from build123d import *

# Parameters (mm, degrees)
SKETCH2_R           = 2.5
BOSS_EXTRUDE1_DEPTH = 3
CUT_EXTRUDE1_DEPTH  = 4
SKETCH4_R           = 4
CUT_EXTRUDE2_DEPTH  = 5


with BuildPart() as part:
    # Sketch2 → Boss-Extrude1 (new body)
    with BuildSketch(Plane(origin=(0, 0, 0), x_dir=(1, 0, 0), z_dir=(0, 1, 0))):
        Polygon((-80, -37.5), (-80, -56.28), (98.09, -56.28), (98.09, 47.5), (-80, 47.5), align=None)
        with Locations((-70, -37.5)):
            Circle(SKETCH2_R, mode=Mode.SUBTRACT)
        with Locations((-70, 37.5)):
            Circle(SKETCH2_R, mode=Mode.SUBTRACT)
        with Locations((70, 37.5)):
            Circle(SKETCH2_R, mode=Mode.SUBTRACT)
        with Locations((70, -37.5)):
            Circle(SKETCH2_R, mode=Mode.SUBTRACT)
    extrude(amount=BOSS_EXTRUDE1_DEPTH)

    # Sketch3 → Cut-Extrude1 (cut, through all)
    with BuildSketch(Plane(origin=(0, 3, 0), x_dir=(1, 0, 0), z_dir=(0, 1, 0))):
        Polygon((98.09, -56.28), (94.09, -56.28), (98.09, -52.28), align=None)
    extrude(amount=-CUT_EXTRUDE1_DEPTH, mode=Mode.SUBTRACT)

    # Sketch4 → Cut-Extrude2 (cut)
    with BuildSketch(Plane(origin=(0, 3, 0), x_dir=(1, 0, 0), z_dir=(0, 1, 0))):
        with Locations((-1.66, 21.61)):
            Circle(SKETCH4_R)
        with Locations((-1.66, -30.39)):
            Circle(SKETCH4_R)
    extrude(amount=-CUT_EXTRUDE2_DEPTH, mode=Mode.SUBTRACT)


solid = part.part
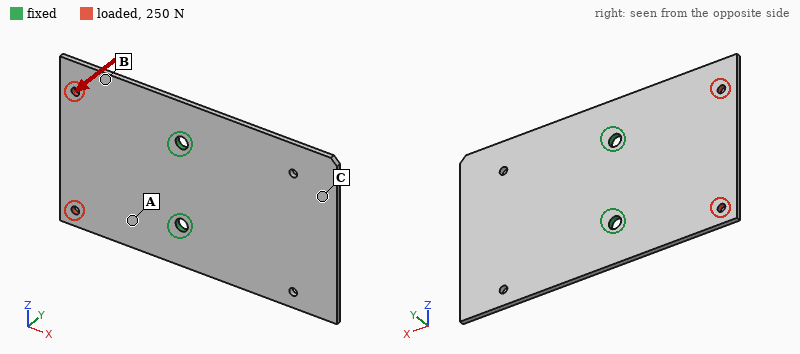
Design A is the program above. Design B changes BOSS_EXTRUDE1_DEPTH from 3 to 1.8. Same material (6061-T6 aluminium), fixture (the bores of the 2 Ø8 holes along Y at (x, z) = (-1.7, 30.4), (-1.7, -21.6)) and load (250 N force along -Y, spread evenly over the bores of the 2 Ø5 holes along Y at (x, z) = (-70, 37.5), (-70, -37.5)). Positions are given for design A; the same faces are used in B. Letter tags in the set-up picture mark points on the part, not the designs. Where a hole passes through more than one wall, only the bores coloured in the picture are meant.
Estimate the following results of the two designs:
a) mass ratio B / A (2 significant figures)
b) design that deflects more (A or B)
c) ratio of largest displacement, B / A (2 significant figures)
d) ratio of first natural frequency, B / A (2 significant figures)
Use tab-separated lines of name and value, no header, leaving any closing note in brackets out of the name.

mass ratio B / A	0.60
design that deflects more	B
ratio of largest displacement, B / A	4.6
ratio of first natural frequency, B / A	0.60
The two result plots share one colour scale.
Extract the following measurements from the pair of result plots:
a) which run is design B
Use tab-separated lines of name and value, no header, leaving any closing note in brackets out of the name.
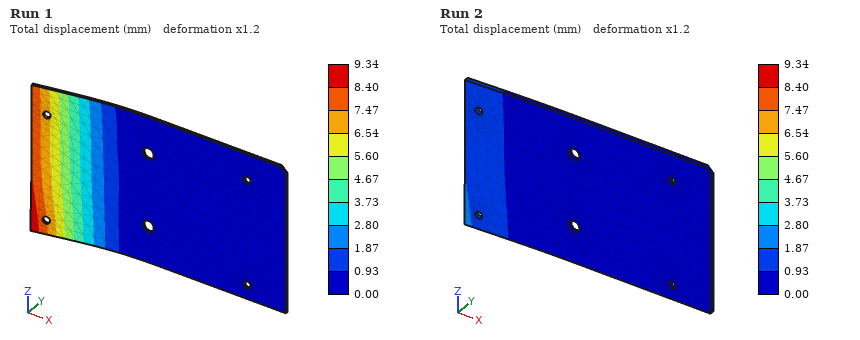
which run is design B	Run 1
